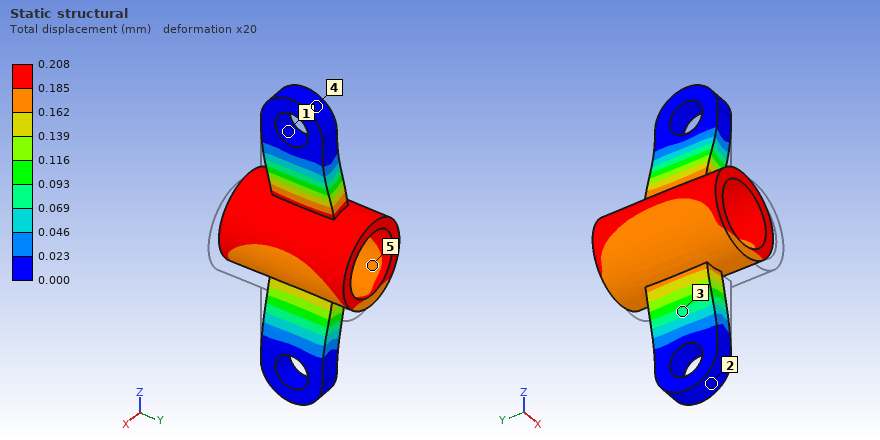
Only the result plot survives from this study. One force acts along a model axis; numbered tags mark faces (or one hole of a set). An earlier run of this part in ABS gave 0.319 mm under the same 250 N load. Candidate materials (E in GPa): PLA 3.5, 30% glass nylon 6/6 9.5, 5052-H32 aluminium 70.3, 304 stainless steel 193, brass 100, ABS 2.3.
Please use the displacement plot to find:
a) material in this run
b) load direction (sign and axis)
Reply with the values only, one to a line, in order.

PLA
-X
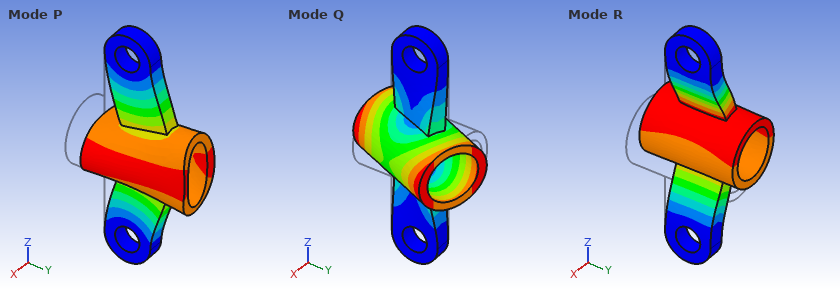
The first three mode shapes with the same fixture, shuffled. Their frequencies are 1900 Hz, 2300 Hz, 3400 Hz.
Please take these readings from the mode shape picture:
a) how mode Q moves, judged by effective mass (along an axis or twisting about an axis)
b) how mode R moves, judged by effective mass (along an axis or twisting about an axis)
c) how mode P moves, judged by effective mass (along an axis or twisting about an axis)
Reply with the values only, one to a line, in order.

twisting about Z
along X
along Y
